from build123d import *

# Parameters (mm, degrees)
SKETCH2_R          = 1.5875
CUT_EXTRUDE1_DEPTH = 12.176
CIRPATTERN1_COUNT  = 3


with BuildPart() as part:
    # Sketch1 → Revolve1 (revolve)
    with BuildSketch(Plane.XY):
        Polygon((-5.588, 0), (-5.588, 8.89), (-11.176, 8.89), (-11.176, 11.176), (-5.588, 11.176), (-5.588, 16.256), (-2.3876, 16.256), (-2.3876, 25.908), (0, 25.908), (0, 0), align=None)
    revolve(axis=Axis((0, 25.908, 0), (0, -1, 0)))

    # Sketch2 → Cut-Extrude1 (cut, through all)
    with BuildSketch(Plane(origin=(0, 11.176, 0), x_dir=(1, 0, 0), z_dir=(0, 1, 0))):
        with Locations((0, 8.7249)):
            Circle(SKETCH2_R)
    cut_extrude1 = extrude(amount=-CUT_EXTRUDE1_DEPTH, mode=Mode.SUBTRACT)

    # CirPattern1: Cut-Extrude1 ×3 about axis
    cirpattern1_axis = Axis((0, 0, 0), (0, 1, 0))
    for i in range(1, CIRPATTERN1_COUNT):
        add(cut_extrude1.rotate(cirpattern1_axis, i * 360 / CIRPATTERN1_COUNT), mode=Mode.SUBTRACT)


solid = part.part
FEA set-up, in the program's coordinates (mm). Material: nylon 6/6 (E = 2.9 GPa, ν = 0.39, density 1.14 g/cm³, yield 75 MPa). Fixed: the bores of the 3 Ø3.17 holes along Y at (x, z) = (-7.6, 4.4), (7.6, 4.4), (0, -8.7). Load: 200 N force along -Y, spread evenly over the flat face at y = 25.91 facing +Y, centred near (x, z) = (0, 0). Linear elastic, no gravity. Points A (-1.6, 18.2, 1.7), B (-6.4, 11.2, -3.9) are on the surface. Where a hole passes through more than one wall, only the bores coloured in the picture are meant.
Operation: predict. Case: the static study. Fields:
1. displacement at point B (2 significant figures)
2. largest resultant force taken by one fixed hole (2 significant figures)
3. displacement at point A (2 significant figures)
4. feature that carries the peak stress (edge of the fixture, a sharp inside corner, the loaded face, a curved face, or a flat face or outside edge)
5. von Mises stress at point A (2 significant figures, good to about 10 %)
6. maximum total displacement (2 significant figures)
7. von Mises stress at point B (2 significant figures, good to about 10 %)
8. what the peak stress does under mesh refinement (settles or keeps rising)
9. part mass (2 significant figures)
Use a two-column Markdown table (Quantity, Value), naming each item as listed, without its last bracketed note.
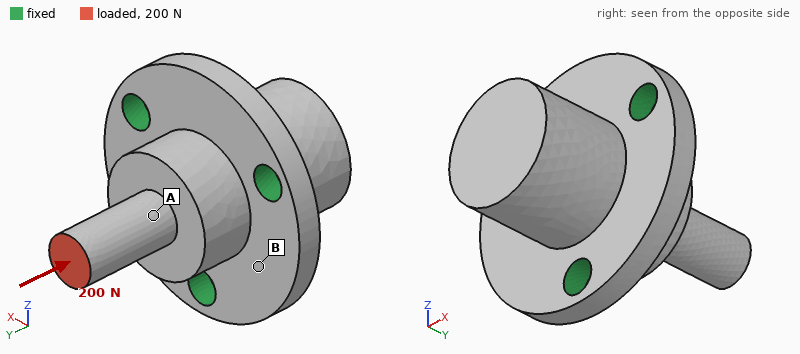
| Quantity | Value |
|---|---|
| displacement at point B | 17 µm |
| largest resultant force taken by one fixed hole | 67 N |
| displacement at point A | 34 µm |
| feature that carries the peak stress | edge of the fixture |
| von Mises stress at point A | 11 MPa |
| maximum total displacement | 64 µm |
| von Mises stress at point B | 2.6 MPa |
| what the peak stress does under mesh refinement | keeps rising |
| part mass | 2.7 g |
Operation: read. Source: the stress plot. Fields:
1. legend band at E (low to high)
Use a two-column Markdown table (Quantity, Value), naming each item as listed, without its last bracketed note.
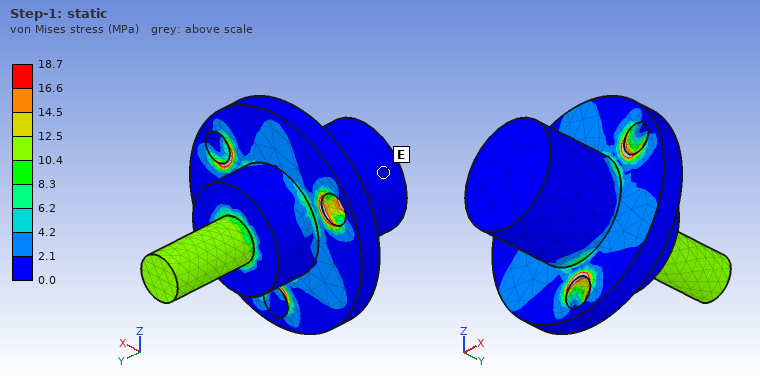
| Quantity | Value |
|---|---|
| legend band at E | 0.0 to 2.1 MPa |
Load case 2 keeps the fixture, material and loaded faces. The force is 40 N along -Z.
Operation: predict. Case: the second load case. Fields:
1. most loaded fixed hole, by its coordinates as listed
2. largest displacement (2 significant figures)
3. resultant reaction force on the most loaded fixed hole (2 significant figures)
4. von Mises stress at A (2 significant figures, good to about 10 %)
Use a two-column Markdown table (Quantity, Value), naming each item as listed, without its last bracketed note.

| Quantity | Value |
|---|---|
| most loaded fixed hole, by its coordinates as listed | (0, -8.7) |
| largest displacement | 0.29 mm |
| resultant reaction force on the most loaded fixed hole | 57 N |
| von Mises stress at A | 21 MPa |
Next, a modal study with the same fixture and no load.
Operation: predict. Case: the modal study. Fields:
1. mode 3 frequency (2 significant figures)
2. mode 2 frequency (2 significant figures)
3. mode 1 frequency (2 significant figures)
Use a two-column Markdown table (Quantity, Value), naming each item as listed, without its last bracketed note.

| Quantity | Value |
|---|---|
| mode 3 frequency | 10 kHz |
| mode 2 frequency | 6900 Hz |
| mode 1 frequency | 6800 Hz |
